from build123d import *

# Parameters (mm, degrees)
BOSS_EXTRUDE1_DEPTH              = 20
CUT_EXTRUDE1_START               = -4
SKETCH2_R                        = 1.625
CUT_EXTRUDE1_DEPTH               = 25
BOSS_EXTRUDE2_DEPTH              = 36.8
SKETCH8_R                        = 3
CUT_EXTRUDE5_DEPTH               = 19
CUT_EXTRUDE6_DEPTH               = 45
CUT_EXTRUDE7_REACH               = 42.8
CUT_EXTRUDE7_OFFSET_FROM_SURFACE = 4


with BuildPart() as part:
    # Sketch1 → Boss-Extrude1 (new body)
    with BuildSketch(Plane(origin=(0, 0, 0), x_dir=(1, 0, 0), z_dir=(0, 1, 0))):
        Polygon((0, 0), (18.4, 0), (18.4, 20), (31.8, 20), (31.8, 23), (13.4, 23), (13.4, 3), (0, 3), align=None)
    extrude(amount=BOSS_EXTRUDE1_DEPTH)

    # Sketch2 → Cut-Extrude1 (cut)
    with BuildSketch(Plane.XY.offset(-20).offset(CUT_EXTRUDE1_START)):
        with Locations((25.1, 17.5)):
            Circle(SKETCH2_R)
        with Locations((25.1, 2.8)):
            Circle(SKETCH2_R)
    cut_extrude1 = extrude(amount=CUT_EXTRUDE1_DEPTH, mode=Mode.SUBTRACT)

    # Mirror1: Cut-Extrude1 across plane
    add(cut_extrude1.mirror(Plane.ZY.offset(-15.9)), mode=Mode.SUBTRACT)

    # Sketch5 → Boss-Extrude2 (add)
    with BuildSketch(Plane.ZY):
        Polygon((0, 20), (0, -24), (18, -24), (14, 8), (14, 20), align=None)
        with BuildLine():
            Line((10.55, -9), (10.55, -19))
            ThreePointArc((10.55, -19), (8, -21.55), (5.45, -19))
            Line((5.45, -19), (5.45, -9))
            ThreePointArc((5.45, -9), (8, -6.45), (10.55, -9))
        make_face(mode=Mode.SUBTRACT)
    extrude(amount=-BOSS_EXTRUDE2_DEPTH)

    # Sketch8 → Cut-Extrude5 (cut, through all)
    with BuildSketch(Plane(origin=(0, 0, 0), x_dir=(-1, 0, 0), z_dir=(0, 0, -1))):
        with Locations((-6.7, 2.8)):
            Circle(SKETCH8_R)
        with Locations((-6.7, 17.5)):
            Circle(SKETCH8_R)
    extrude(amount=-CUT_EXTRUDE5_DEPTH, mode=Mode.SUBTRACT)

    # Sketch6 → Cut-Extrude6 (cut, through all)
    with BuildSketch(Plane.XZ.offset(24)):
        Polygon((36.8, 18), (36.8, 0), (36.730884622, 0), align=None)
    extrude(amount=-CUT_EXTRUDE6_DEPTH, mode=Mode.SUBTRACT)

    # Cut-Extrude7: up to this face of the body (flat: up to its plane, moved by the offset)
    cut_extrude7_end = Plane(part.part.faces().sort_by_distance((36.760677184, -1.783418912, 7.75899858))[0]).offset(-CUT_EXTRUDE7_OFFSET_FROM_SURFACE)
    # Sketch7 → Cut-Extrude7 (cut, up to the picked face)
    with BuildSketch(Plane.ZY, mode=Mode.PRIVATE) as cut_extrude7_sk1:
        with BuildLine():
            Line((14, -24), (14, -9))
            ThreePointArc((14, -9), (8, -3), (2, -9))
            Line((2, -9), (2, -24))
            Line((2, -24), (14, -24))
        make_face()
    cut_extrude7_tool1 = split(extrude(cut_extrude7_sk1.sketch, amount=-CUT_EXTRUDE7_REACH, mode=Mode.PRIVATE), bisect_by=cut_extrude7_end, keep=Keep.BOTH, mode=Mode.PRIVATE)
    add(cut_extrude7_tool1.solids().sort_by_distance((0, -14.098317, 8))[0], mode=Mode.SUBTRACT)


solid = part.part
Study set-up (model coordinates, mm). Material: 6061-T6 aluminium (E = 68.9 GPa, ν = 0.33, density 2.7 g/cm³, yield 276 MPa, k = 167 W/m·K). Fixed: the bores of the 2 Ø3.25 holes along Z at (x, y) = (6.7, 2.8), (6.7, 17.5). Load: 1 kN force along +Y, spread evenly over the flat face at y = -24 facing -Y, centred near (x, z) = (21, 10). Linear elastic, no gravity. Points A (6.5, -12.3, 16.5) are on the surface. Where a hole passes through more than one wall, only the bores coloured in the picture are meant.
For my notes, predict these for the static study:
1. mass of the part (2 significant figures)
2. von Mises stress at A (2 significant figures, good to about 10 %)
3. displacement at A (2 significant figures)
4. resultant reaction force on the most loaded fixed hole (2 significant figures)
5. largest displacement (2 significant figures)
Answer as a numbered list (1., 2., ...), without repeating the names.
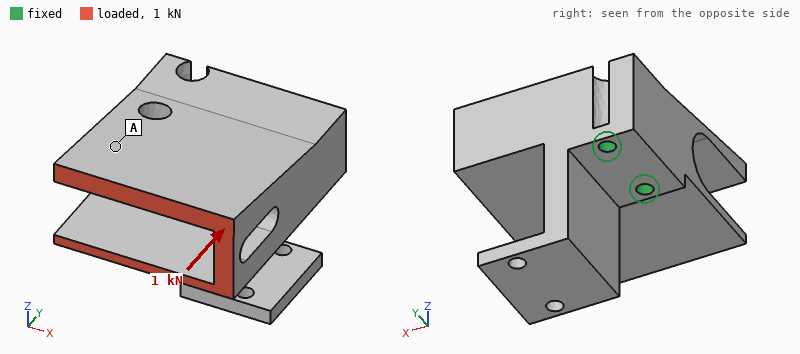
1. 54 g
2. 9.5 MPa
3. 24 µm
4. 1.3 kN
5. 46 µm
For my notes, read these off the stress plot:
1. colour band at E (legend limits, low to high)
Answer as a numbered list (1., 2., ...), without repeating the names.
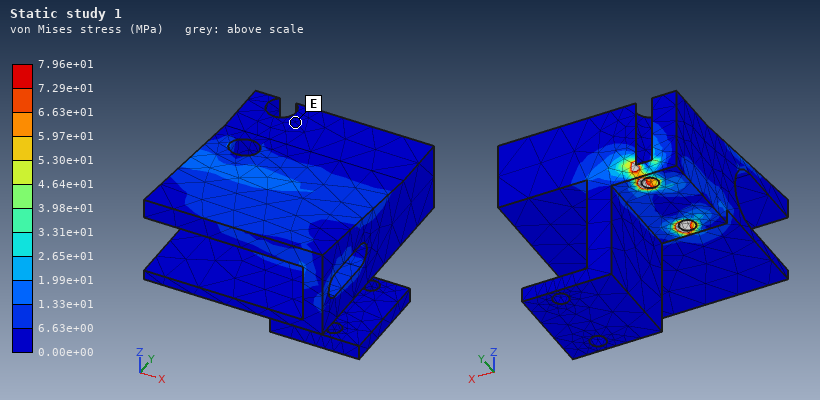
1. 0.00e+00 to 6.63e+00 MPa
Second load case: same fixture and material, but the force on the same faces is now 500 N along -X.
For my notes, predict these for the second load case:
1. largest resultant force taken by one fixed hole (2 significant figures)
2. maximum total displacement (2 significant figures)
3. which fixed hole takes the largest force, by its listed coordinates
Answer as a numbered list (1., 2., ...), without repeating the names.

1. 1.3 kN
2. 80 µm
3. (6.7, 2.8)
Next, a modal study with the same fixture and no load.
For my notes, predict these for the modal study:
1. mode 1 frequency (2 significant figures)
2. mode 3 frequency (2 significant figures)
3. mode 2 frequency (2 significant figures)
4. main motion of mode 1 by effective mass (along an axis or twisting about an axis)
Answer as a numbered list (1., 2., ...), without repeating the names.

1. 2000 Hz
2. 5200 Hz
3. 4500 Hz
4. along Z
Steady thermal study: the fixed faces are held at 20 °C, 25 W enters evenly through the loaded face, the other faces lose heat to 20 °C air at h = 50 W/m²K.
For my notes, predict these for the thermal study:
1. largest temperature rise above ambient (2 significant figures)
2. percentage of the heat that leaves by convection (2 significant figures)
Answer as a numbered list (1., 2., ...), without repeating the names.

1. 27 K
2. 20 %
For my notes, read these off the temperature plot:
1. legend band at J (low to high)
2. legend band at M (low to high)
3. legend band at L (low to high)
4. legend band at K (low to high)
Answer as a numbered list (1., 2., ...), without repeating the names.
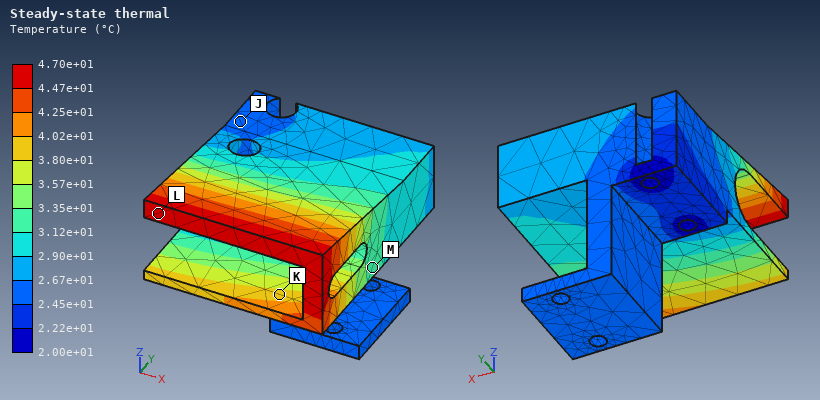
1. 2.45e+01 to 2.67e+01 °C
2. 3.12e+01 to 3.35e+01 °C
3. 4.47e+01 to 4.70e+01 °C
4. 3.80e+01 to 4.02e+01 °C
